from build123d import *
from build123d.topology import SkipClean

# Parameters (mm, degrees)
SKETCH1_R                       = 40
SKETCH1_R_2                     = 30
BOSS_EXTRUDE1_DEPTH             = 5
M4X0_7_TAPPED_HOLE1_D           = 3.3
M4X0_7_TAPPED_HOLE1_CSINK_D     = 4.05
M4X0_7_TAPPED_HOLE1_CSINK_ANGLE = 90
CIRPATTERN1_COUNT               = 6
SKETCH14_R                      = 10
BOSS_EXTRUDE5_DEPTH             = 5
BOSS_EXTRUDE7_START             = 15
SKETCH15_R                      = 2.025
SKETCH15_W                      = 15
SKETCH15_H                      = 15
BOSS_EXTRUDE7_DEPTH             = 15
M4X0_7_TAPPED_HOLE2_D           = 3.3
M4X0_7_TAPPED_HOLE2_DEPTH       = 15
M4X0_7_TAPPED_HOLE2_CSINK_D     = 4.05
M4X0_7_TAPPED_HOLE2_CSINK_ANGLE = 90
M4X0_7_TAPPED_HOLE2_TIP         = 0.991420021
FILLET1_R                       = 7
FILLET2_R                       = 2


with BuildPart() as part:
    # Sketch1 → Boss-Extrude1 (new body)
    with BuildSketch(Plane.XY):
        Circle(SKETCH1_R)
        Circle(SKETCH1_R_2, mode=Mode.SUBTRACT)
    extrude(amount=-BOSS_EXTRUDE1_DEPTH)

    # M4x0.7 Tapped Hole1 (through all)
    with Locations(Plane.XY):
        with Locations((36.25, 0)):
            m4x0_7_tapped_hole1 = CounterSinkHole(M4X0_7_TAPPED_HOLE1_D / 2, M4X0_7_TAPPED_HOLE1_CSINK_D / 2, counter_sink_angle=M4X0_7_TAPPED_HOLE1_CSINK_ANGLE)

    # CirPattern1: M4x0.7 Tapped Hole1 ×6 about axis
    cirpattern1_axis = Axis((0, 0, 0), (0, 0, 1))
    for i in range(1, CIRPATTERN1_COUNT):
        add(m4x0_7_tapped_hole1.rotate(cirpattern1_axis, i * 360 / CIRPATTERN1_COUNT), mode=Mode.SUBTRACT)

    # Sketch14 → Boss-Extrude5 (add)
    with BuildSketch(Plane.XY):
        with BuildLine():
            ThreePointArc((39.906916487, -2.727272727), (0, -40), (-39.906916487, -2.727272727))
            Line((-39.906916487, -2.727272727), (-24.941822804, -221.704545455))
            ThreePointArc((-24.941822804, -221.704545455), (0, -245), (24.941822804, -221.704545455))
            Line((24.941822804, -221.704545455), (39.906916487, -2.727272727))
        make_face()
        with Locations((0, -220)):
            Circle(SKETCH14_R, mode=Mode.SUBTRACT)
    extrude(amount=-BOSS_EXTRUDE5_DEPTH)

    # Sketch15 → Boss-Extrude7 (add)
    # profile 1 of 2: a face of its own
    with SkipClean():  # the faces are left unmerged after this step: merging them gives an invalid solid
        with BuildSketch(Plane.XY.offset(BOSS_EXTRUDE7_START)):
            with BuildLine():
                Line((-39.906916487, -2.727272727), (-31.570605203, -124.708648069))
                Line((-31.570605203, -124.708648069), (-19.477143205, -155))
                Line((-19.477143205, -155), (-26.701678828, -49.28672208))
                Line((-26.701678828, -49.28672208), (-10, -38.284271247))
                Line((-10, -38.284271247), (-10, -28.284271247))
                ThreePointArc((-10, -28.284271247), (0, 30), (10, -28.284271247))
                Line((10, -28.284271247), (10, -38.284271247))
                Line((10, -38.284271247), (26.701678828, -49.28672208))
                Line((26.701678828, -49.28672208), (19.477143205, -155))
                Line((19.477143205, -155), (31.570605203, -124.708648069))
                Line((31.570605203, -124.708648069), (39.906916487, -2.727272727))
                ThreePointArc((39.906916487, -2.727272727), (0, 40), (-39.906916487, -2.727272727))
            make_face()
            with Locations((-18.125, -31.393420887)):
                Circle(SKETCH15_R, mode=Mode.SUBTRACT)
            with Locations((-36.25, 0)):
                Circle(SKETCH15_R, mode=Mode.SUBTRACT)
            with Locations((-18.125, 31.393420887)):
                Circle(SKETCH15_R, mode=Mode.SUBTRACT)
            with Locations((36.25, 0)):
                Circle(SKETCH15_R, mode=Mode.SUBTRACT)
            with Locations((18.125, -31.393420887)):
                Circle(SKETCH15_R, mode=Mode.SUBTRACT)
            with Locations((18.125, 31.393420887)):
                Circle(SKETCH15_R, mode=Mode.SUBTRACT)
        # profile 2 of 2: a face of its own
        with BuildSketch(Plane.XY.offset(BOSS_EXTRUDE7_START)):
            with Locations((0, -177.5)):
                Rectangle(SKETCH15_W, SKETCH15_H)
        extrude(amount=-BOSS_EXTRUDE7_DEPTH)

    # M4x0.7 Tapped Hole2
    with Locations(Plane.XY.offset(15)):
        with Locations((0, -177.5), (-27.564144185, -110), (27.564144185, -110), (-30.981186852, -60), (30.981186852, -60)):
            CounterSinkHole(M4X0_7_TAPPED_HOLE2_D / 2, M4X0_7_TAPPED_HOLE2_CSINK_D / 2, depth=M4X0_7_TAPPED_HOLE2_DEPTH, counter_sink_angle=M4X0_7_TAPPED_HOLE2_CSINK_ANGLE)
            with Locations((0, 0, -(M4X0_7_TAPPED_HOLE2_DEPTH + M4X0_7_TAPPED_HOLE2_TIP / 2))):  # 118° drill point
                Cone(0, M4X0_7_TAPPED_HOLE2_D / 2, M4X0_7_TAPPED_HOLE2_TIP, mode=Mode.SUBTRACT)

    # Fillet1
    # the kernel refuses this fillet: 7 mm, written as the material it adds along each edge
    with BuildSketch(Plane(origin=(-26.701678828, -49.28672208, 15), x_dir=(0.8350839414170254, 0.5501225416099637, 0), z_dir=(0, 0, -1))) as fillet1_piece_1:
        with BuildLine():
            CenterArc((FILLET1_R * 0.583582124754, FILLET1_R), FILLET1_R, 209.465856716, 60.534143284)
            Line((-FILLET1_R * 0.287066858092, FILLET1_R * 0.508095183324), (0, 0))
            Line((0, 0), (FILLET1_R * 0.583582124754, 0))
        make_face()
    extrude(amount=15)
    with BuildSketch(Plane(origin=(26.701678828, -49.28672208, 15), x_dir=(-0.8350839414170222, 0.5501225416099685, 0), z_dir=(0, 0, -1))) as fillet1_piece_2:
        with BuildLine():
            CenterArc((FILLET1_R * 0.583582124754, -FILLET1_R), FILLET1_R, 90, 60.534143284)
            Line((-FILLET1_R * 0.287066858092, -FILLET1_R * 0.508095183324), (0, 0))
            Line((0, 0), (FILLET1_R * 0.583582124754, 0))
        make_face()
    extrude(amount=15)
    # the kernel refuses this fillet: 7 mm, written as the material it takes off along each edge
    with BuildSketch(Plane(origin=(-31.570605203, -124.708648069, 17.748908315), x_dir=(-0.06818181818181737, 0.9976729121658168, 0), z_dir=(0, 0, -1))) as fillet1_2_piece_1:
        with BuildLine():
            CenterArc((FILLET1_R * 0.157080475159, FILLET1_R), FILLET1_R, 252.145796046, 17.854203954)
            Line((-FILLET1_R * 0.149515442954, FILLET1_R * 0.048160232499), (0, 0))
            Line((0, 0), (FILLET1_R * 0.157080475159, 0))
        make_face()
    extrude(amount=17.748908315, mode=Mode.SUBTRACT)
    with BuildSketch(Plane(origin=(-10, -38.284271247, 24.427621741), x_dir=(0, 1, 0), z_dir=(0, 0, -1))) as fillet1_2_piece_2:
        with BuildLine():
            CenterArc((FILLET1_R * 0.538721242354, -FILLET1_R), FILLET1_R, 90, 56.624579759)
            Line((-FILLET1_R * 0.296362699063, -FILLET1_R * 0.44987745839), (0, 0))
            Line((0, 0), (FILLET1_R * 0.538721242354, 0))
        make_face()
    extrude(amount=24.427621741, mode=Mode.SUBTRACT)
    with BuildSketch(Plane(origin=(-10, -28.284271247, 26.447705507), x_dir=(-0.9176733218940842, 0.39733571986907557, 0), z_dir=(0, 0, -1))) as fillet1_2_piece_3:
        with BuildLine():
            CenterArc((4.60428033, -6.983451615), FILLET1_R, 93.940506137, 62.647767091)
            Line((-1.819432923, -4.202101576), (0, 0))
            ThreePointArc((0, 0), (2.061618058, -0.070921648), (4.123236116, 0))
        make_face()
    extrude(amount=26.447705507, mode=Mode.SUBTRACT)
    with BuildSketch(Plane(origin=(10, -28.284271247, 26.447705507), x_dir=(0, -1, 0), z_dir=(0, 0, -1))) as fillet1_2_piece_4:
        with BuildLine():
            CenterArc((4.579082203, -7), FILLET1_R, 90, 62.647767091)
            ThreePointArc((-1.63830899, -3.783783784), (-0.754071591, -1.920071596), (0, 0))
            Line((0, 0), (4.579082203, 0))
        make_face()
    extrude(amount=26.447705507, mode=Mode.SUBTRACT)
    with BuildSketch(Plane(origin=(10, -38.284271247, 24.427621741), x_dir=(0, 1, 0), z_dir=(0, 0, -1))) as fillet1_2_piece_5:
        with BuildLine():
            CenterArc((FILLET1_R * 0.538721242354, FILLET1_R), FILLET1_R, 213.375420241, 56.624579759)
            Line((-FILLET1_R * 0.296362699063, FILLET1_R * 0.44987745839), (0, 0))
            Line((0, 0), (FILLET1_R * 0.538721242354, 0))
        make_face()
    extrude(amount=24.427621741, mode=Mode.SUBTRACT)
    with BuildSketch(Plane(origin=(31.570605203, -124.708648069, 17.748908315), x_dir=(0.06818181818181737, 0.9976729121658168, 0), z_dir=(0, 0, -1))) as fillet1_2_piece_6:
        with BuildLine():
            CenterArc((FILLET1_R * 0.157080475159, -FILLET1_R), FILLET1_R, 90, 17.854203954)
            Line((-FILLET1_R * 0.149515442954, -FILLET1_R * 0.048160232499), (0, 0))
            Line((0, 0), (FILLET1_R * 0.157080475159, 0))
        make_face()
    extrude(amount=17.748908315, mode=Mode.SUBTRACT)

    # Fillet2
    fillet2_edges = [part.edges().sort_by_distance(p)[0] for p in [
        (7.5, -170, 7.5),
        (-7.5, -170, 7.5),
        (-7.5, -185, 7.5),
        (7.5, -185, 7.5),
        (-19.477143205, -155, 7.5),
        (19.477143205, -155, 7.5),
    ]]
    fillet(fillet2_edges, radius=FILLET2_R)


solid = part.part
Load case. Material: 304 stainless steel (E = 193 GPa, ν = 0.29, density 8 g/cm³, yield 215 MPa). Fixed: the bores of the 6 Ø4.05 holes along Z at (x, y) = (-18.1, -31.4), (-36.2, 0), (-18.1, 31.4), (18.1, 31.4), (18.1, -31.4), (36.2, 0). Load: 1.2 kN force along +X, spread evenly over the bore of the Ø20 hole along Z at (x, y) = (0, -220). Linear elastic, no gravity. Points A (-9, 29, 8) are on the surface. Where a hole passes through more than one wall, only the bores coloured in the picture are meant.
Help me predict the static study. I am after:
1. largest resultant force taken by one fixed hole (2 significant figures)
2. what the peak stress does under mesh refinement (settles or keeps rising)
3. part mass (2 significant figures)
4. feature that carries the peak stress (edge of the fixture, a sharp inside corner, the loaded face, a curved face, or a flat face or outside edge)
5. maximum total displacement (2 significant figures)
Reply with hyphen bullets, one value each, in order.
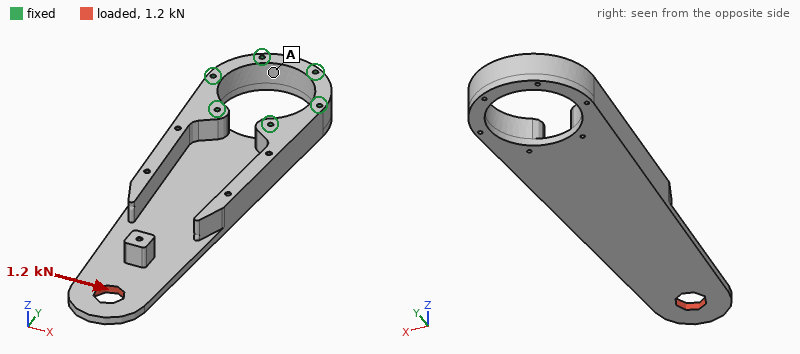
- 2.1 kN
- keeps rising
- 1.2 kg
- edge of the fixture
- 99 µm
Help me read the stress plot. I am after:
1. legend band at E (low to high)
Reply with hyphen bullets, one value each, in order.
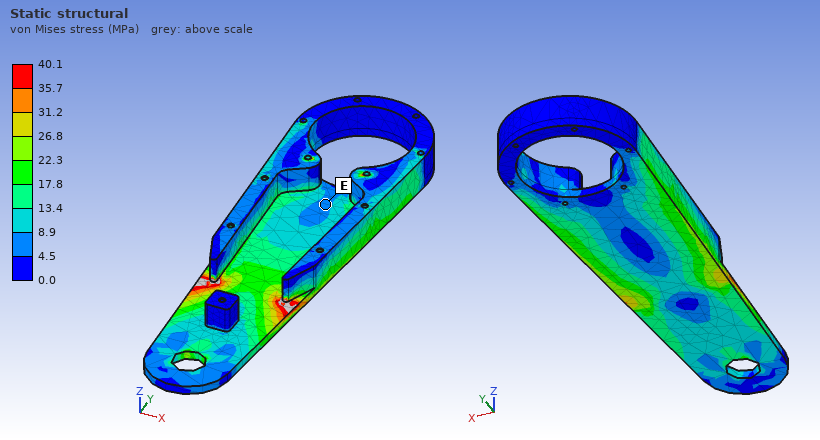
- 4.5 to 8.9 MPa
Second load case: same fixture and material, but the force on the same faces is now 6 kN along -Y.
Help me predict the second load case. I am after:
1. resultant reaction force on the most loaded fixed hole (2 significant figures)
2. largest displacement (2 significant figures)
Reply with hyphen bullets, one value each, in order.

- 2.2 kN
- 0.14 mm
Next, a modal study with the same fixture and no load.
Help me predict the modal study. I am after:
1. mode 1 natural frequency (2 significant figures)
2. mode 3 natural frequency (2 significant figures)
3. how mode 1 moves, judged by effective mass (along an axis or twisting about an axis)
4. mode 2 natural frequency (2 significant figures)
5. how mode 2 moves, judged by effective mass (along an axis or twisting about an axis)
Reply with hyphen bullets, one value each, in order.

- 350 Hz
- 1200 Hz
- along Z
- 1100 Hz
- along Z
